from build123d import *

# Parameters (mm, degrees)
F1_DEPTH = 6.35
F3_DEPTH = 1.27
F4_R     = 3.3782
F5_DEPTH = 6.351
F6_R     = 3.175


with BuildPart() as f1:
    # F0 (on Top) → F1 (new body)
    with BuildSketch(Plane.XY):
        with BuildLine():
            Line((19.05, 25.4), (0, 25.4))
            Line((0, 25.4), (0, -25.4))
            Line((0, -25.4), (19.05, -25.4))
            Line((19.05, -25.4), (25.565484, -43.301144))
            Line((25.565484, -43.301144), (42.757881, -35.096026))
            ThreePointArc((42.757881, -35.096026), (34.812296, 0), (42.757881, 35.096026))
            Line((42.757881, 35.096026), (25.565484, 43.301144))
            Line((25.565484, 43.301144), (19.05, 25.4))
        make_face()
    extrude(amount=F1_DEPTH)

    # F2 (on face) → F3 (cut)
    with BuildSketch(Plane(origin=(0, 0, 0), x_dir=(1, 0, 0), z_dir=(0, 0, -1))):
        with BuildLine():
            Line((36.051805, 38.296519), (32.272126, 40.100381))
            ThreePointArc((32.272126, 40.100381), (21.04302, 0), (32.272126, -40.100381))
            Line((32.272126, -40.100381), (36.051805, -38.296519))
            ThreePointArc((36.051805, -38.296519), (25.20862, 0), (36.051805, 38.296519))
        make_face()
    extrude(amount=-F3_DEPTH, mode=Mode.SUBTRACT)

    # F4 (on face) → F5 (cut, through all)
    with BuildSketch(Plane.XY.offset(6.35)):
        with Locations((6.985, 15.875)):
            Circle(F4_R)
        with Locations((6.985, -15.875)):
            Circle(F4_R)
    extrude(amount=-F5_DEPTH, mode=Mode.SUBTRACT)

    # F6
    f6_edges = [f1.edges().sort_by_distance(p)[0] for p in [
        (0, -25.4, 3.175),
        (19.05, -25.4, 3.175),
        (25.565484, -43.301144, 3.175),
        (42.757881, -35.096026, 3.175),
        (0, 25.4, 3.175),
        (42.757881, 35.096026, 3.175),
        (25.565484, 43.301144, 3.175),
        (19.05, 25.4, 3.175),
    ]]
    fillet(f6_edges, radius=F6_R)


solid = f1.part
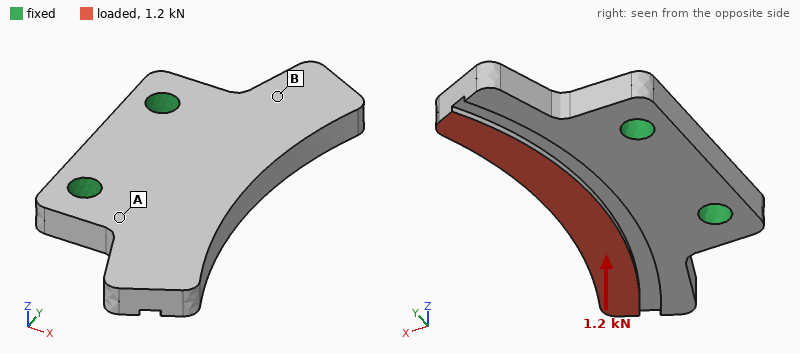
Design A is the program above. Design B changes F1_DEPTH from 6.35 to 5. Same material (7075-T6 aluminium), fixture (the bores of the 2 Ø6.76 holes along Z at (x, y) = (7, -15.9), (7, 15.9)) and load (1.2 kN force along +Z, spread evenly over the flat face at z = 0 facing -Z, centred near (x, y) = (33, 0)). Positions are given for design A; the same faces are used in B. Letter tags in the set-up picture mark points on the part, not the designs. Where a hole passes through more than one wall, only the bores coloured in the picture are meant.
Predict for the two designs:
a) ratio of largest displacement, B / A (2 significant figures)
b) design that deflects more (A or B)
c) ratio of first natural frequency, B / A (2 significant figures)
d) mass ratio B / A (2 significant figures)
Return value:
2.0
B
0.81
0.78
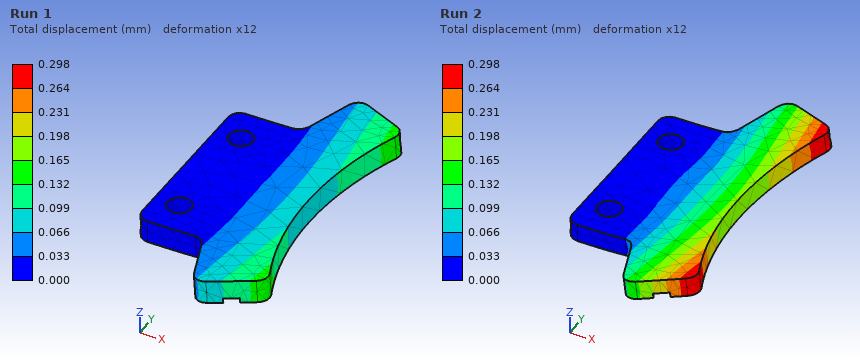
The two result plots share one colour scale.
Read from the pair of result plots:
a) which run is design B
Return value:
Run 2
